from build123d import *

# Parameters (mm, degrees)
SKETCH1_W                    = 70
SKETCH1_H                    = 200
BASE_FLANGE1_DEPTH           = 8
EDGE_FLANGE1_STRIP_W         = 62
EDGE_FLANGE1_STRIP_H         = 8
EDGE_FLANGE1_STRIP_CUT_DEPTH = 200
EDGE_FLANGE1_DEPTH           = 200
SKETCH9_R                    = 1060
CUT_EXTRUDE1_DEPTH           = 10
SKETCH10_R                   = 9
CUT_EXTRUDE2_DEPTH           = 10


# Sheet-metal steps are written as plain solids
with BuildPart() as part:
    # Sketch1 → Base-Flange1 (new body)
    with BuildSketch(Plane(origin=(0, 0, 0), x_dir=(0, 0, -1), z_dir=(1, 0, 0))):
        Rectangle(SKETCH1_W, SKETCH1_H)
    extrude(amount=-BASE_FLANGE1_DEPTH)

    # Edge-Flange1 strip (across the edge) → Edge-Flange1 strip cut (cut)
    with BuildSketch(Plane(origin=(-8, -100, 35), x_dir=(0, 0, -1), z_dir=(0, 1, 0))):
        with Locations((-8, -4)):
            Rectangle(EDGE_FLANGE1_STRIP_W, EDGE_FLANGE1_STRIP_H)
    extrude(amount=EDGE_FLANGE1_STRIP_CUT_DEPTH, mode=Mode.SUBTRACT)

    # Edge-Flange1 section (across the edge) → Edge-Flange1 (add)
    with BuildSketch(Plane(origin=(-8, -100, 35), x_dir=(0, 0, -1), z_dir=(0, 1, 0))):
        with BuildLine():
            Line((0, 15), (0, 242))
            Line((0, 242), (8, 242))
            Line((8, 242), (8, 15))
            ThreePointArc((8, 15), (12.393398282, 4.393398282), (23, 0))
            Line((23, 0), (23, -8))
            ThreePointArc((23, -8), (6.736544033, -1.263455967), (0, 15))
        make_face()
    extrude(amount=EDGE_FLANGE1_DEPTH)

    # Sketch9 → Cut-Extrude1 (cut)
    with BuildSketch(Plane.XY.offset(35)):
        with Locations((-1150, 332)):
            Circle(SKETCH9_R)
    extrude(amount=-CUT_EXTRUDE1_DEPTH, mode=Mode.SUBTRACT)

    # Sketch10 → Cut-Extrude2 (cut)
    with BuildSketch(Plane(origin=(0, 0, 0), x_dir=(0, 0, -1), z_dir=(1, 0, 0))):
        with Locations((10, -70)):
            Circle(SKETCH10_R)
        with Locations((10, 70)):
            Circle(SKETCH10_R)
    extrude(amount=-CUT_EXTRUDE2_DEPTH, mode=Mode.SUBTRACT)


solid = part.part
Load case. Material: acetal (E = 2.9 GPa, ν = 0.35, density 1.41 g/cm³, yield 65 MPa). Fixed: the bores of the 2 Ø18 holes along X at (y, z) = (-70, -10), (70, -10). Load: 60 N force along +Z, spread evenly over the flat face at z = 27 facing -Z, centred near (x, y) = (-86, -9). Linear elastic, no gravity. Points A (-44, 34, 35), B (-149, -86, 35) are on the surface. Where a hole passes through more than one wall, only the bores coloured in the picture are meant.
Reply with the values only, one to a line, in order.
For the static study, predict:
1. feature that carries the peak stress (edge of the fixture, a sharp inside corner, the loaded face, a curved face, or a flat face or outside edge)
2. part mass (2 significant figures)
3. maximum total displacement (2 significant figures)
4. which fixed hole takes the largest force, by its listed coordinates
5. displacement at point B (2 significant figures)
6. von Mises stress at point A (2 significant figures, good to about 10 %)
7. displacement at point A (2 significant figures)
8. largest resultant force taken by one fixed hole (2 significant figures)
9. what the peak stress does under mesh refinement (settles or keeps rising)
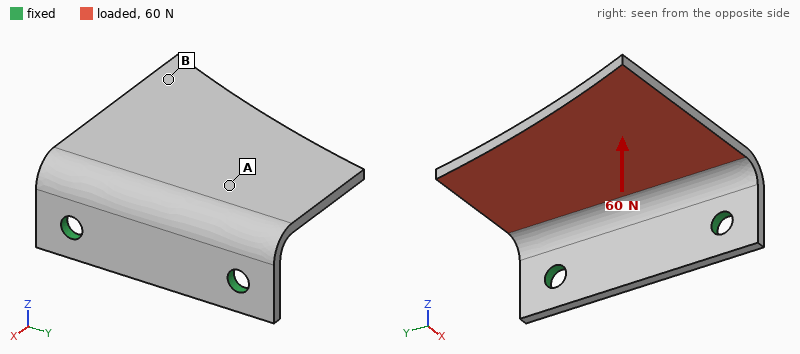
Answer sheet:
edge of the fixture
440 g
2.6 mm
(-70, -10)
2.0 mm
1.0 MPa
0.41 mm
35 N
keeps rising
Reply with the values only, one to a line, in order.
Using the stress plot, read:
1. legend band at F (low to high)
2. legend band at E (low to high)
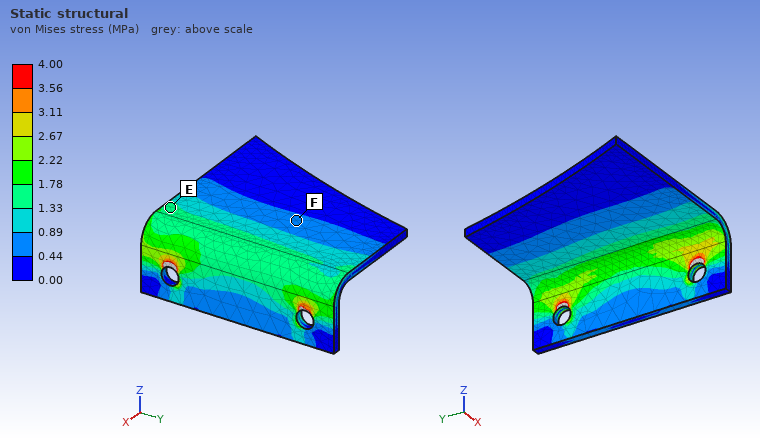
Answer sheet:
0.44 to 0.89 MPa
1.33 to 1.78 MPa
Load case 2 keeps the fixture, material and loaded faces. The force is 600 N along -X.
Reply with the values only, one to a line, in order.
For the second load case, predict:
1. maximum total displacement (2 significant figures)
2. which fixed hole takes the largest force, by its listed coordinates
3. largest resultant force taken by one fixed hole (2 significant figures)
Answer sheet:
2.1 mm
(-70, -10)
340 N
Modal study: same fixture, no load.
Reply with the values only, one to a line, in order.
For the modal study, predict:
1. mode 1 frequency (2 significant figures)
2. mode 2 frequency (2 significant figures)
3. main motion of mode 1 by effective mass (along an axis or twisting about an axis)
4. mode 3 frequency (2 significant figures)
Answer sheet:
64 Hz
150 Hz
along Z
280 Hz
